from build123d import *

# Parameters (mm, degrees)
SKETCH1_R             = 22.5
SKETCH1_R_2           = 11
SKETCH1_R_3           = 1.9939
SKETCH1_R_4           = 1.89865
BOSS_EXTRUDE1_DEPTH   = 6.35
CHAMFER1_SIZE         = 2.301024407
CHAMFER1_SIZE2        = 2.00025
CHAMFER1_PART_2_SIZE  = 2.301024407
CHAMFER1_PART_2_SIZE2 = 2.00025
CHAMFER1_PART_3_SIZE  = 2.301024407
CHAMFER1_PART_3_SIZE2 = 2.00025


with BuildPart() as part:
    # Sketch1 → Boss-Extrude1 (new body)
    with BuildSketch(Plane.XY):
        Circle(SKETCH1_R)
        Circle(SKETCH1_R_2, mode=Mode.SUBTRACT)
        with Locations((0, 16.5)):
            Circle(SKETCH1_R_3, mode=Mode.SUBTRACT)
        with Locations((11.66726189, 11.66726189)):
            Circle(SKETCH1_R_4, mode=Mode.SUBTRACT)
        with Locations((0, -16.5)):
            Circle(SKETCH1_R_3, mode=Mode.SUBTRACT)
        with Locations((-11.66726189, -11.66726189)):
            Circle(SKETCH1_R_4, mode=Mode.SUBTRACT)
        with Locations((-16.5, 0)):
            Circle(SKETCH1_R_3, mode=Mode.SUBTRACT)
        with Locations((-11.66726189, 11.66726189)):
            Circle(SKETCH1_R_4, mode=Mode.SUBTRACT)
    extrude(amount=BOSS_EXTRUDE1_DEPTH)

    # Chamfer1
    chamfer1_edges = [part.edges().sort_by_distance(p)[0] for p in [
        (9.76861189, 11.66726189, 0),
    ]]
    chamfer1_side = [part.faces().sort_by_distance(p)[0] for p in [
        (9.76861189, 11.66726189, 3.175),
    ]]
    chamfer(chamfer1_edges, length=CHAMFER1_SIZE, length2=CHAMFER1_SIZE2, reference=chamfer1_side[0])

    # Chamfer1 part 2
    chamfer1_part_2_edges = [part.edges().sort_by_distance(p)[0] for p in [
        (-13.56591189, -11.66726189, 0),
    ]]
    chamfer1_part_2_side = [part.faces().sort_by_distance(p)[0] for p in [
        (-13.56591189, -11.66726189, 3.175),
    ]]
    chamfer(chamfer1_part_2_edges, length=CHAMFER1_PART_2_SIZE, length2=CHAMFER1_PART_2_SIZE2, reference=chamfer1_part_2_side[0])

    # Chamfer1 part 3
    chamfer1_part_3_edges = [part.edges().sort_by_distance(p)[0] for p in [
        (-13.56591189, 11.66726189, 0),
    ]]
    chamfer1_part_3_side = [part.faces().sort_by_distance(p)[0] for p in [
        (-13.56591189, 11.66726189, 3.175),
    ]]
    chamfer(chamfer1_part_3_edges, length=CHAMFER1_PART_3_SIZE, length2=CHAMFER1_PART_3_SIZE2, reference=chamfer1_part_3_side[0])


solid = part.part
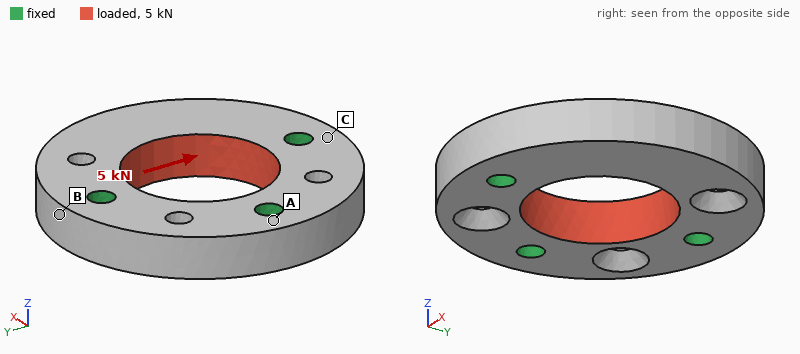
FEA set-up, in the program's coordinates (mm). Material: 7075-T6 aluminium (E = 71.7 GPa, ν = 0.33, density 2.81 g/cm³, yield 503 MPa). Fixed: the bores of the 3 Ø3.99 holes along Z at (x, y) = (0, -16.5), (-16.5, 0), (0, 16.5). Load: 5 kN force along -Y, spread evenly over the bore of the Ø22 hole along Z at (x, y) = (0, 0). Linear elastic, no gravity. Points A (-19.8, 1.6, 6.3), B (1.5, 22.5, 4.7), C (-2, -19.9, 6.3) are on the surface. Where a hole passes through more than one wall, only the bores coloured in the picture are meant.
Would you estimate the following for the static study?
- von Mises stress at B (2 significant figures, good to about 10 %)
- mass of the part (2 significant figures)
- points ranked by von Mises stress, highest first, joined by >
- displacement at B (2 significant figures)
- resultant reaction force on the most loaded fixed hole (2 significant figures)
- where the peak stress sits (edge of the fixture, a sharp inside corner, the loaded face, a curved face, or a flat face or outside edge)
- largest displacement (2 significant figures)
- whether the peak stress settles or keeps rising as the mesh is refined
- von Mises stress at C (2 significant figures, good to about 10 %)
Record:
24 MPa
20 g
B > C > A
2.1 µm
2.0 kN
edge of the fixture
12 µm
keeps rising
14 MPa
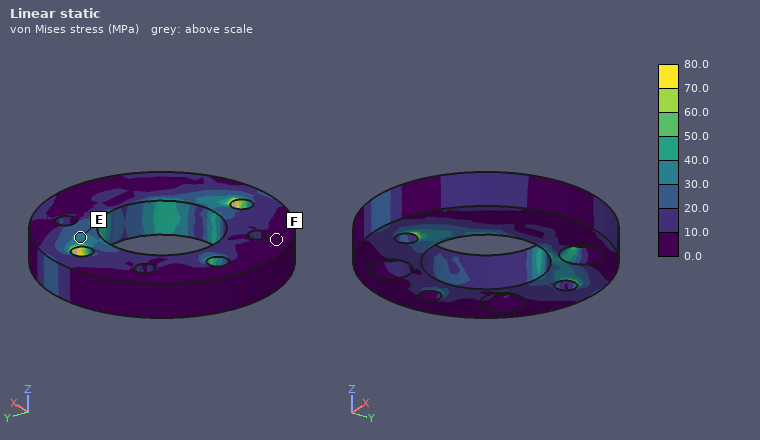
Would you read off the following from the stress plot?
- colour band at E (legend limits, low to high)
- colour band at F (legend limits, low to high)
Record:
30.0 to 40.0 MPa
0.0 to 10.0 MPa
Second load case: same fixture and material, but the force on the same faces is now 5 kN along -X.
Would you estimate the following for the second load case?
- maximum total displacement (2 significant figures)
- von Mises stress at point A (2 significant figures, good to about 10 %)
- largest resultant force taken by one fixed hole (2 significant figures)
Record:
8.3 µm
6.1 MPa
1.9 kN
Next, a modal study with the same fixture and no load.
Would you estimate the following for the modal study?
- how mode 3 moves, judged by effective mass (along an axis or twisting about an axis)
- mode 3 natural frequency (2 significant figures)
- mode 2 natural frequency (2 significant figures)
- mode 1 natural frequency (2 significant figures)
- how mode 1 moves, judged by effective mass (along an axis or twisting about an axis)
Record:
along Y
24 kHz
22 kHz
8900 Hz
along Z
